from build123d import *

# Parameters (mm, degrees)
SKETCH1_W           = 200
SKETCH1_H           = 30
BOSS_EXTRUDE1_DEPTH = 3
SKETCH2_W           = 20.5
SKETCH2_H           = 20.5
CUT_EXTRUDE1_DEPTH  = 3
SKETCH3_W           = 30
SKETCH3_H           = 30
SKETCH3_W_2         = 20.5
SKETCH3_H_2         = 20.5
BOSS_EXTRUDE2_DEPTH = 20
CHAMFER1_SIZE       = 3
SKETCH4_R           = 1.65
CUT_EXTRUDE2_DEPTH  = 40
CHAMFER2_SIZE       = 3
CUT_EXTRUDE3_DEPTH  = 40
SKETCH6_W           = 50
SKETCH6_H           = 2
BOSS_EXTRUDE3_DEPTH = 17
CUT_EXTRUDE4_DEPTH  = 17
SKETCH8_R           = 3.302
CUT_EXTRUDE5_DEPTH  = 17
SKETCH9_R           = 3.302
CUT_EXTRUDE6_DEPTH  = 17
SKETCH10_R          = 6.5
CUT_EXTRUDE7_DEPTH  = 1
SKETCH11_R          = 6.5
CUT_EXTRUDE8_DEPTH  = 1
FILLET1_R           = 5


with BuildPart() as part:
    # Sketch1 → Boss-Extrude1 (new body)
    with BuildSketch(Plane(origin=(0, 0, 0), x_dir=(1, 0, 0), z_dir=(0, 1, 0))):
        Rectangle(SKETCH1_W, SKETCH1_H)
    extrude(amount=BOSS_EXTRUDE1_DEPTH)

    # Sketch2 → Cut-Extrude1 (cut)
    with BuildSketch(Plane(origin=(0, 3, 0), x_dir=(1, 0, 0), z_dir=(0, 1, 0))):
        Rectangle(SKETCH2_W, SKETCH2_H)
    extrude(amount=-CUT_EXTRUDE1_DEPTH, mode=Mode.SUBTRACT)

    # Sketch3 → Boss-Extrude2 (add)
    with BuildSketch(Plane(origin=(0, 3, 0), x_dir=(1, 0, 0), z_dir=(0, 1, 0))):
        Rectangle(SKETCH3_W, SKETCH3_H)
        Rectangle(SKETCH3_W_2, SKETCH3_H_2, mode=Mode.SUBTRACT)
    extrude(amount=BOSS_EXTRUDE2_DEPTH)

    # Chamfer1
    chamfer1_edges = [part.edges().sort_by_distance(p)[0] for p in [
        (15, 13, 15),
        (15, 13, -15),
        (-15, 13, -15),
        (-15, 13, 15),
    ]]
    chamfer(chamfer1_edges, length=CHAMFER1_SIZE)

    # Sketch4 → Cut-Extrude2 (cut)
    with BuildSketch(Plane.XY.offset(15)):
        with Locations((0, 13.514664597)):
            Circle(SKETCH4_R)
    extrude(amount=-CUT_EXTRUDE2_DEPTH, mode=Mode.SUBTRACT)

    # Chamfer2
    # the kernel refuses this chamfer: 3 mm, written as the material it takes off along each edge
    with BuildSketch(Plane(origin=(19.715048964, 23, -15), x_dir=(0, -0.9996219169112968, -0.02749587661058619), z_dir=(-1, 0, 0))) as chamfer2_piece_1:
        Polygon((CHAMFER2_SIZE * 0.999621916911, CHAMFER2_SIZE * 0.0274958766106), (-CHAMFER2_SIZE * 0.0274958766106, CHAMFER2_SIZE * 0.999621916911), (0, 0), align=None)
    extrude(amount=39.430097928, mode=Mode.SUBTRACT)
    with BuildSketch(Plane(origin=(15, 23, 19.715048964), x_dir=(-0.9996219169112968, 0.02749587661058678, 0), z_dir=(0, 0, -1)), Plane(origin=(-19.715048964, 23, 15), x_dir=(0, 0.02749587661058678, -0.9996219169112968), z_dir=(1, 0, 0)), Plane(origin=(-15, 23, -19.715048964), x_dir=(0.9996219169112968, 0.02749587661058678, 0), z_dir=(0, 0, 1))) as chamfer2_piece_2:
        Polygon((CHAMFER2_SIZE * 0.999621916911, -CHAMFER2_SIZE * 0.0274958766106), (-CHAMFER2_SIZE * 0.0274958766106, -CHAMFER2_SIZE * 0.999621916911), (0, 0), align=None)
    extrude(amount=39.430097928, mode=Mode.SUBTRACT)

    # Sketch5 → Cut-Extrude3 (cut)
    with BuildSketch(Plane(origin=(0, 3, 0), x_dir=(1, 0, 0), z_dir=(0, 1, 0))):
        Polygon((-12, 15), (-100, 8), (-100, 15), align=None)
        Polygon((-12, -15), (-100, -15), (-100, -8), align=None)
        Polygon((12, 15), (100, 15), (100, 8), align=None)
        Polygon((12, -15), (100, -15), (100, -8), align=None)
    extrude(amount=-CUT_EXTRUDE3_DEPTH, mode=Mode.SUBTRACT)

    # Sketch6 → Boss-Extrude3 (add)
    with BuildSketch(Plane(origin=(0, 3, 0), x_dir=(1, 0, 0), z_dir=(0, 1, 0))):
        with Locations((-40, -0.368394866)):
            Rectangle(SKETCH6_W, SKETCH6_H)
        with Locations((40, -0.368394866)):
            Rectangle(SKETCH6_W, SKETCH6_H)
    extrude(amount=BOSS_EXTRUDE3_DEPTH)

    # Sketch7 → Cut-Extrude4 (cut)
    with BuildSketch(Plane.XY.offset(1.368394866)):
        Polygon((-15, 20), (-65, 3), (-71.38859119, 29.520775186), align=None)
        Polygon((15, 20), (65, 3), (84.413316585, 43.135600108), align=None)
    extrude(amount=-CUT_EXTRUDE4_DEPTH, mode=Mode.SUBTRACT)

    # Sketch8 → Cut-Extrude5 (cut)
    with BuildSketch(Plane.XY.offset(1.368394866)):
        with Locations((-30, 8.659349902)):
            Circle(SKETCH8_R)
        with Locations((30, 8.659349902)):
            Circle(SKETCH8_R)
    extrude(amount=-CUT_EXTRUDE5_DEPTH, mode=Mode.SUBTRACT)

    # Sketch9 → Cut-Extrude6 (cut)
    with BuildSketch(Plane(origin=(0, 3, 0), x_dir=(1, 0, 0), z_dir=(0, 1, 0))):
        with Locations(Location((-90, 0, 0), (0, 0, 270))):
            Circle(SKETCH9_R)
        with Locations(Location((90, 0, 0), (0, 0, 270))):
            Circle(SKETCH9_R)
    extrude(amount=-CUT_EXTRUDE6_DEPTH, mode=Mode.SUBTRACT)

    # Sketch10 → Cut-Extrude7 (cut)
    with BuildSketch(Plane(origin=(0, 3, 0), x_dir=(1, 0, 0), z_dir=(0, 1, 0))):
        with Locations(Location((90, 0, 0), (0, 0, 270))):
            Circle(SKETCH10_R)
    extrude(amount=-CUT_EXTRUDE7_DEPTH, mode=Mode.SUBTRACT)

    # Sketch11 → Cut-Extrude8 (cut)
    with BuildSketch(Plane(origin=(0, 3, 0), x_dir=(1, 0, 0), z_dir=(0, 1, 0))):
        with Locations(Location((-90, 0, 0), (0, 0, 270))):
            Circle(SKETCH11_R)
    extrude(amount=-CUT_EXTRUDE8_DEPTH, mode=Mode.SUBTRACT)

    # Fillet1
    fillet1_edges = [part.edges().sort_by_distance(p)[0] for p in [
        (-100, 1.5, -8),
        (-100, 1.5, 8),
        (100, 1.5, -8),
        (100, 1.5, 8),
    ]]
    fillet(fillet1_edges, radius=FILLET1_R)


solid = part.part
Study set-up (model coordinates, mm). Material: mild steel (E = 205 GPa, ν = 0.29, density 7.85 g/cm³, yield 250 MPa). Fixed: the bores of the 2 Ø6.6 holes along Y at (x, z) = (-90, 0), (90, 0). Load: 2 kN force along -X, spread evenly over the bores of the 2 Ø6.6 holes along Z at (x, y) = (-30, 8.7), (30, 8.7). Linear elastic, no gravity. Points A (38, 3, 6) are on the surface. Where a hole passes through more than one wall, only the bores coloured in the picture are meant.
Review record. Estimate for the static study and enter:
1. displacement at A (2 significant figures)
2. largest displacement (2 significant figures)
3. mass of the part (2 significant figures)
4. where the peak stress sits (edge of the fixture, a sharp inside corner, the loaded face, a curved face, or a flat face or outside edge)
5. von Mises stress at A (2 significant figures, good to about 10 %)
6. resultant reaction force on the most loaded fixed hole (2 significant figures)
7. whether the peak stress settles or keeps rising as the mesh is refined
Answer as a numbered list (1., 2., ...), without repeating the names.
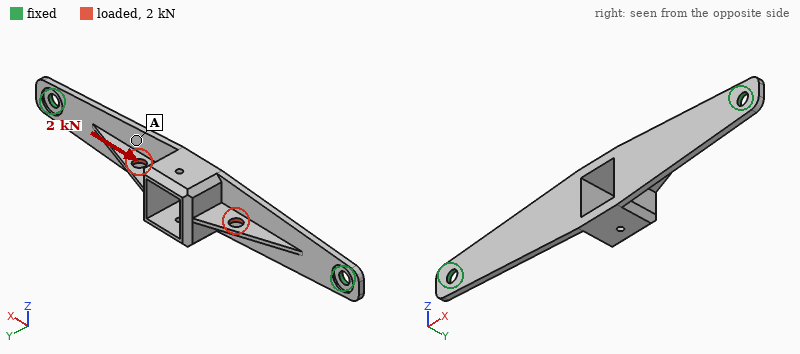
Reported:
1. 24 µm
2. 30 µm
3. 180 g
4. edge of the fixture
5. 11 MPa
6. 1.0 kN
7. keeps rising
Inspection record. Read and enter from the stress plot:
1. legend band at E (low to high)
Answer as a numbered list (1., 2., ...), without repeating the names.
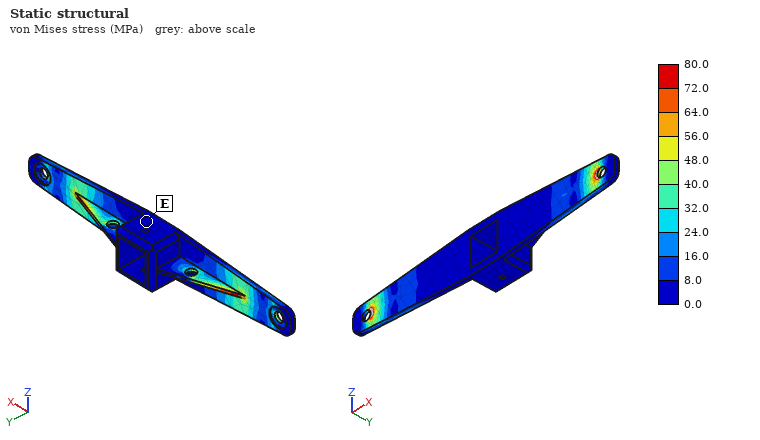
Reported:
1. 0.0 to 8.0 MPa
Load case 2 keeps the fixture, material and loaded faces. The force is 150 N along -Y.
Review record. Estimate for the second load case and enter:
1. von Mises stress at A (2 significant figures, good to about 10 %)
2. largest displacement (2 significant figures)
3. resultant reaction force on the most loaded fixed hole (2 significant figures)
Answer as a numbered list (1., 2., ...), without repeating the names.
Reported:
1. 5.2 MPa
2. 60 µm
3. 220 N
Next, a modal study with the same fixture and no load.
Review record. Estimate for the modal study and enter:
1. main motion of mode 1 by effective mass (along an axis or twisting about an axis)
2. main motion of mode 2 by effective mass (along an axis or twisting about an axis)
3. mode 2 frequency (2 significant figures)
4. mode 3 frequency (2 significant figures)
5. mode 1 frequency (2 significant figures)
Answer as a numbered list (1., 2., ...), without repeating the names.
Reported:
1. along Y
2. along Z
3. 700 Hz
4. 1800 Hz
5. 660 Hz
